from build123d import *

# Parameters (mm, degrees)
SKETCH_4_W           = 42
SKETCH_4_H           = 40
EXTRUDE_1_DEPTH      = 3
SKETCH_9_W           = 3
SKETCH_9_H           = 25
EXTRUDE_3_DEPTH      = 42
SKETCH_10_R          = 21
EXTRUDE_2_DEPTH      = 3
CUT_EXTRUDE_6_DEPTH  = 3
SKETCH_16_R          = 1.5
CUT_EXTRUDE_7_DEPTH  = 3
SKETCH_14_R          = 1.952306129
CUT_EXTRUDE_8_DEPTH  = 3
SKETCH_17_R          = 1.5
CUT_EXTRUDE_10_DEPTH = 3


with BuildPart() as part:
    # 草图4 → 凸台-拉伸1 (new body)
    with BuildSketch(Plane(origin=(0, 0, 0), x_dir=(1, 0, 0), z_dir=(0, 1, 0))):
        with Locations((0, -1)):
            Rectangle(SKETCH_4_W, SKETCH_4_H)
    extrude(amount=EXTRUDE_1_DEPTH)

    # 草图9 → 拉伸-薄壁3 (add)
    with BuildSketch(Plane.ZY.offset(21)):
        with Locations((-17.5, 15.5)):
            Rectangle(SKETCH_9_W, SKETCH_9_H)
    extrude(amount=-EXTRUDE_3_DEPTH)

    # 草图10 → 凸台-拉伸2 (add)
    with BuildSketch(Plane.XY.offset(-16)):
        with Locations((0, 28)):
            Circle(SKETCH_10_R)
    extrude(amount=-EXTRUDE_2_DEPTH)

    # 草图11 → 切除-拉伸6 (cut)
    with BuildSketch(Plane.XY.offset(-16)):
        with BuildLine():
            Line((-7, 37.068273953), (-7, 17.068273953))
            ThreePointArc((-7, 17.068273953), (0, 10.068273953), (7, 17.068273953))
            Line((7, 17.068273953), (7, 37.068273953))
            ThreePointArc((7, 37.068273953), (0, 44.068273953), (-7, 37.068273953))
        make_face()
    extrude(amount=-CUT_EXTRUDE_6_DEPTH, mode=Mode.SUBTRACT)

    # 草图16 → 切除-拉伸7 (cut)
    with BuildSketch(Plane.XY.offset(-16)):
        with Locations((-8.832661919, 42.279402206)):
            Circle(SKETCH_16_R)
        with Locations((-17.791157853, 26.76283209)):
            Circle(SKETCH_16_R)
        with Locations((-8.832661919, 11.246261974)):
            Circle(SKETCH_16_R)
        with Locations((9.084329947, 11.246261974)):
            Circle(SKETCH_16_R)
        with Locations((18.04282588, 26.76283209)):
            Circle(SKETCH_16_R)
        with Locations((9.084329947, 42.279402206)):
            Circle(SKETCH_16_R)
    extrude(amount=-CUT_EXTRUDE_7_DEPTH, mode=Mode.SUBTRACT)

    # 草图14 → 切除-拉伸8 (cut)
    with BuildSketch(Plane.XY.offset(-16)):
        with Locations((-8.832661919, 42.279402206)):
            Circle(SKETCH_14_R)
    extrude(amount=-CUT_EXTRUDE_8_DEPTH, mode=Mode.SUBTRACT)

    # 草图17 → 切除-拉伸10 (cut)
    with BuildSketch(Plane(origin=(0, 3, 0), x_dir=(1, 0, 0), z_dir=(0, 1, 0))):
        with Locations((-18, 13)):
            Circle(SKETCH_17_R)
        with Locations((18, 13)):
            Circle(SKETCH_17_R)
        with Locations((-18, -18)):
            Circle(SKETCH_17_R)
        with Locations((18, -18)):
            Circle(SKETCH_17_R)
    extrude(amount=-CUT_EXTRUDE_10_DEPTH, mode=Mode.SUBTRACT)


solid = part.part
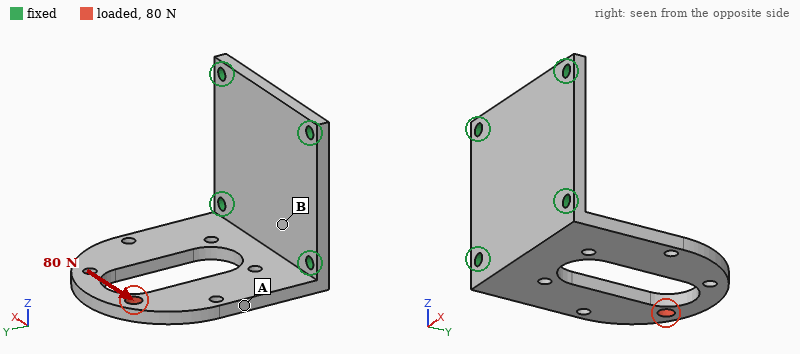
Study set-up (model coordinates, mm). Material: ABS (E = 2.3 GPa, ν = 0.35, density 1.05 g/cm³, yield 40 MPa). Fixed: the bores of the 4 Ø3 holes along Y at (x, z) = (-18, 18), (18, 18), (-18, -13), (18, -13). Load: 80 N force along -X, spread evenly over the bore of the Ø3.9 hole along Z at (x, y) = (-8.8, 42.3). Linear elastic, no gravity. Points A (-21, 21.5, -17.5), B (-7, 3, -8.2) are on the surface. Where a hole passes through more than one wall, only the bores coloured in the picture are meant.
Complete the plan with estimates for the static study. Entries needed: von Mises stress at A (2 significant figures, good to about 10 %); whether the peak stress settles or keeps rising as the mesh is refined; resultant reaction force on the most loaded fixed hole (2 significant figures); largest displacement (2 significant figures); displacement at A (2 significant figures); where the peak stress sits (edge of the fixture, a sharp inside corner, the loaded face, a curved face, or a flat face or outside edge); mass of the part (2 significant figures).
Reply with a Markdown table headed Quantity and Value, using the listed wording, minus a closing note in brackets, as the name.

| Quantity | Value |
|---|---|
| von Mises stress at A | 5.2 MPa |
| whether the peak stress settles or keeps rising as the mesh is refined | keeps rising |
| resultant reaction force on the most loaded fixed hole | 100 N |
| largest displacement | 0.45 mm |
| displacement at A | 0.23 mm |
| where the peak stress sits | edge of the fixture |
| mass of the part | 9.2 g |
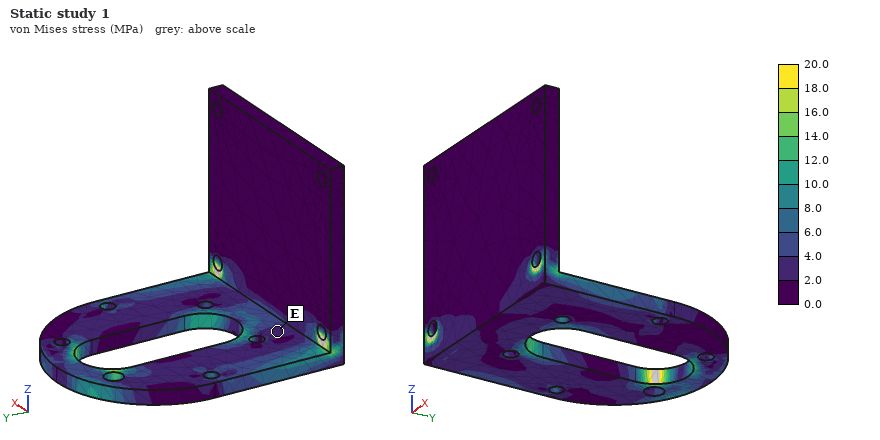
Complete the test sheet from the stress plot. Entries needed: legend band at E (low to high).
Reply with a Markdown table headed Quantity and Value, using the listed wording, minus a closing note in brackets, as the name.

| Quantity | Value |
|---|---|
| legend band at E | 2.0 to 4.0 MPa |
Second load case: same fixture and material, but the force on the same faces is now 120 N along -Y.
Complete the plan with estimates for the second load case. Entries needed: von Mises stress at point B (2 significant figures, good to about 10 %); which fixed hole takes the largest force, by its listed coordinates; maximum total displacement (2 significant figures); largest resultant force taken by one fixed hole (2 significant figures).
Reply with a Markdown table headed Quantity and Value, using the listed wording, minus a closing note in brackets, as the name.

| Quantity | Value |
|---|---|
| von Mises stress at point B | 1.6 MPa |
| which fixed hole takes the largest force, by its listed coordinates | (-18, -13) |
| maximum total displacement | 0.38 mm |
| largest resultant force taken by one fixed hole | 93 N |
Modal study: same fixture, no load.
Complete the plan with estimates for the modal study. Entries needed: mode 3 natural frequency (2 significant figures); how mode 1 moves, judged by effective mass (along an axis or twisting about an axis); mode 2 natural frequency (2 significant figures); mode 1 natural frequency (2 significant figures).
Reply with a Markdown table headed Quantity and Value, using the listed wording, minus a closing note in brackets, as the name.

| Quantity | Value |
|---|---|
| mode 3 natural frequency | 1800 Hz |
| how mode 1 moves, judged by effective mass | along Z |
| mode 2 natural frequency | 850 Hz |
| mode 1 natural frequency | 350 Hz |
